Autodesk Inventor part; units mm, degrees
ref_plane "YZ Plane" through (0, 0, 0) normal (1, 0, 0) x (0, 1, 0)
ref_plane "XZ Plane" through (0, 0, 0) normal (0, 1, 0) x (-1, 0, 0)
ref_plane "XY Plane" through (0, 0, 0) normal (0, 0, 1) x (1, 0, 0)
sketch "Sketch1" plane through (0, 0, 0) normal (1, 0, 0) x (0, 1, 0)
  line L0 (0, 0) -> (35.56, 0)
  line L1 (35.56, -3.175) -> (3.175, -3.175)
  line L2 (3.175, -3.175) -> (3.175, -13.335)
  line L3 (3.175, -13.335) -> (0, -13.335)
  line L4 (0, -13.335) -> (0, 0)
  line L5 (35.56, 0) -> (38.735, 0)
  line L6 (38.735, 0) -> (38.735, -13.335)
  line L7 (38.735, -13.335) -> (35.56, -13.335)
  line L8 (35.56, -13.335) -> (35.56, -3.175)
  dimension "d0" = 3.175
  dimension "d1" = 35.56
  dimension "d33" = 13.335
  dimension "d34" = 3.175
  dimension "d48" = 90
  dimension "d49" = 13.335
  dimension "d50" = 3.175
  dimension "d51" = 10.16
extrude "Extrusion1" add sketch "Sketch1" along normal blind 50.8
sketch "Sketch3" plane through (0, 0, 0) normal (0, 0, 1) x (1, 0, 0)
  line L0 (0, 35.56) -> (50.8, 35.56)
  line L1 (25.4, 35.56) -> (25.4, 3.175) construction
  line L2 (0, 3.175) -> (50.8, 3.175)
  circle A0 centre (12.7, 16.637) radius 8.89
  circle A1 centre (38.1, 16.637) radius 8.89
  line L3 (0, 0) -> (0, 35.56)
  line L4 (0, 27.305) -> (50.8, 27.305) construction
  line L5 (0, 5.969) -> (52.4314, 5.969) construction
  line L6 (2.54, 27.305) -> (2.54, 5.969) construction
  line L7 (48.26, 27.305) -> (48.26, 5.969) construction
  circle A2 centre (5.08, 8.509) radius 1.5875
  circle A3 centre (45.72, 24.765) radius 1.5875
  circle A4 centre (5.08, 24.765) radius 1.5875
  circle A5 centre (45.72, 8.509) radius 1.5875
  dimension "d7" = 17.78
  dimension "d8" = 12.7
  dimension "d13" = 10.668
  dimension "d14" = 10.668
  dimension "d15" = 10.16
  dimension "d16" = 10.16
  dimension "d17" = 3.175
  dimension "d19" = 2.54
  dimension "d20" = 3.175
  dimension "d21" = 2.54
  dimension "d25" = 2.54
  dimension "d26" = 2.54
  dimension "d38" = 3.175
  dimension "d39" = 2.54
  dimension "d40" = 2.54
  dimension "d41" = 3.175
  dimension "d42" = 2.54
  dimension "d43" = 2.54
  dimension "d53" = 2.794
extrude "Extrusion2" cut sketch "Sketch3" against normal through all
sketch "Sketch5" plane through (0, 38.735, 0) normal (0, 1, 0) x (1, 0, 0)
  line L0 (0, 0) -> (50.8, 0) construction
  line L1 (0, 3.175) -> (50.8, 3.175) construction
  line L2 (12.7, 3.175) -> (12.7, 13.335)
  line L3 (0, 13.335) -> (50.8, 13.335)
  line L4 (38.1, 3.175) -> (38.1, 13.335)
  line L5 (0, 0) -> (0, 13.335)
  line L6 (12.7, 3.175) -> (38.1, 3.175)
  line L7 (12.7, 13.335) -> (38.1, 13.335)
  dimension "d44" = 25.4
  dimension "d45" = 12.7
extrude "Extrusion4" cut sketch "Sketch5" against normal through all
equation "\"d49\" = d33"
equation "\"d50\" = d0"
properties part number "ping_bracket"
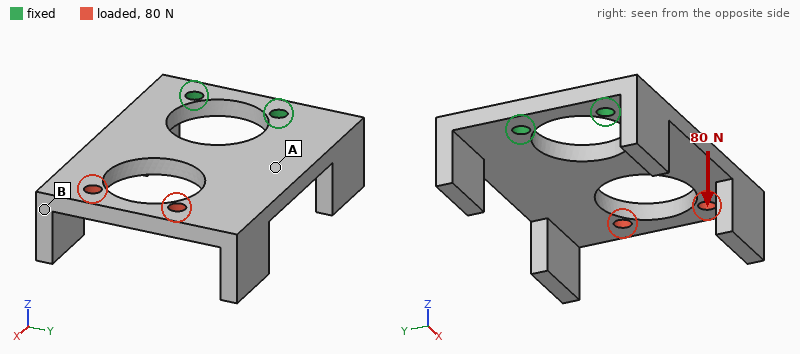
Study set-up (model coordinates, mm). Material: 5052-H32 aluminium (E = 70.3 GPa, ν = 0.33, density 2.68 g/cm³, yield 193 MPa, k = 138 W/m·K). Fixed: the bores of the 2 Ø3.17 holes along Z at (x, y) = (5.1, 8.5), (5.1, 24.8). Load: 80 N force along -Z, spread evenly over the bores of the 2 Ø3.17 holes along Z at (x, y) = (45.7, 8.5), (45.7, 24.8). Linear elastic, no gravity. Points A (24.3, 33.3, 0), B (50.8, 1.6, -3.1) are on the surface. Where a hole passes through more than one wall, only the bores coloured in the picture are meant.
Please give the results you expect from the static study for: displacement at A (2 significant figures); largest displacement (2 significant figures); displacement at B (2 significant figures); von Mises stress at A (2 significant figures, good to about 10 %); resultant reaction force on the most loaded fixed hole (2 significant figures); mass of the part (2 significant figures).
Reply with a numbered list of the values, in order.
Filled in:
1. 0.13 mm
2. 0.52 mm
3. 0.49 mm
4. 35 MPa
5. 44 N
6. 17 g
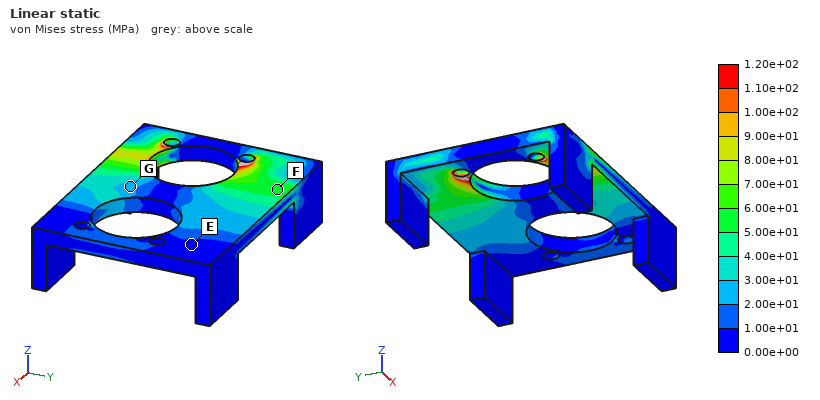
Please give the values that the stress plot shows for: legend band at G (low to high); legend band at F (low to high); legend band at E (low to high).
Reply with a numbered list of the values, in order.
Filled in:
1. 2.00e+01 to 3.00e+01 MPa
2. 5.00e+01 to 6.00e+01 MPa
3. 0.00e+00 to 1.00e+01 MPa
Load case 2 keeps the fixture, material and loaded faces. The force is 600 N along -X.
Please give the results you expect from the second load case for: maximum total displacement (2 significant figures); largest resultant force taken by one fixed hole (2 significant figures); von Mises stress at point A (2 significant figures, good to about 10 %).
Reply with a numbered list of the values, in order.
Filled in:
1. 13 µm
2. 300 N
3. 6.8 MPa
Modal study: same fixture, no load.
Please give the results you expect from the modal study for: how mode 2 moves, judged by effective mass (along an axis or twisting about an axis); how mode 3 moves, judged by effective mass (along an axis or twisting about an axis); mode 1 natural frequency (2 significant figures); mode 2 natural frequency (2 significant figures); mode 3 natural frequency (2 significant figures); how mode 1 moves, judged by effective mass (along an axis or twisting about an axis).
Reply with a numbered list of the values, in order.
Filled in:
1. twisting about X
2. along Y
3. 890 Hz
4. 1900 Hz
5. 4000 Hz
6. along Z
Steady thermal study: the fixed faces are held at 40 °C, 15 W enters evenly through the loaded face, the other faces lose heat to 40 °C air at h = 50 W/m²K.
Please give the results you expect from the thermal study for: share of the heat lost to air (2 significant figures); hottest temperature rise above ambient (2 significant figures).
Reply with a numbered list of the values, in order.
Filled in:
1. 38 %
2. 55 K
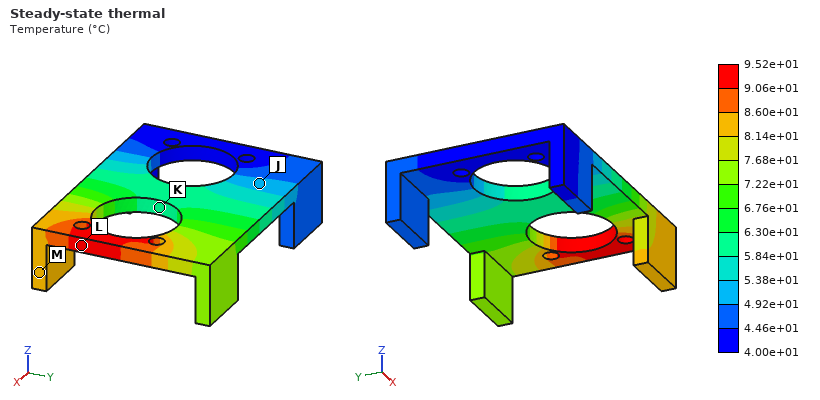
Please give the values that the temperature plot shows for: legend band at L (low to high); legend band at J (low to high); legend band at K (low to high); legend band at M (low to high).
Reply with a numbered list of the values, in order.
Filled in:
1. 9.06e+01 to 9.52e+01 °C
2. 4.92e+01 to 5.38e+01 °C
3. 5.84e+01 to 6.30e+01 °C
4. 8.14e+01 to 8.60e+01 °C
